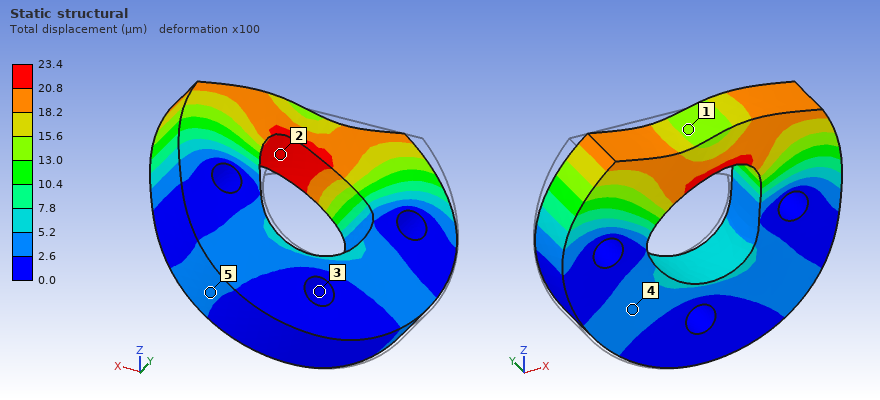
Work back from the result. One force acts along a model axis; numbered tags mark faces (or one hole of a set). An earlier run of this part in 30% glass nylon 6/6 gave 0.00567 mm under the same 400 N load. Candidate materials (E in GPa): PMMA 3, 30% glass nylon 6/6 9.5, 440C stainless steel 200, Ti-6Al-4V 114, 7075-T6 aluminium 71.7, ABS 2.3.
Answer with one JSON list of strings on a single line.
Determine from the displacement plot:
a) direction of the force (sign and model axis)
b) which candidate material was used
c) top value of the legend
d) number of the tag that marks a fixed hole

["+X", "ABS", "23.4 µm", "3"]
